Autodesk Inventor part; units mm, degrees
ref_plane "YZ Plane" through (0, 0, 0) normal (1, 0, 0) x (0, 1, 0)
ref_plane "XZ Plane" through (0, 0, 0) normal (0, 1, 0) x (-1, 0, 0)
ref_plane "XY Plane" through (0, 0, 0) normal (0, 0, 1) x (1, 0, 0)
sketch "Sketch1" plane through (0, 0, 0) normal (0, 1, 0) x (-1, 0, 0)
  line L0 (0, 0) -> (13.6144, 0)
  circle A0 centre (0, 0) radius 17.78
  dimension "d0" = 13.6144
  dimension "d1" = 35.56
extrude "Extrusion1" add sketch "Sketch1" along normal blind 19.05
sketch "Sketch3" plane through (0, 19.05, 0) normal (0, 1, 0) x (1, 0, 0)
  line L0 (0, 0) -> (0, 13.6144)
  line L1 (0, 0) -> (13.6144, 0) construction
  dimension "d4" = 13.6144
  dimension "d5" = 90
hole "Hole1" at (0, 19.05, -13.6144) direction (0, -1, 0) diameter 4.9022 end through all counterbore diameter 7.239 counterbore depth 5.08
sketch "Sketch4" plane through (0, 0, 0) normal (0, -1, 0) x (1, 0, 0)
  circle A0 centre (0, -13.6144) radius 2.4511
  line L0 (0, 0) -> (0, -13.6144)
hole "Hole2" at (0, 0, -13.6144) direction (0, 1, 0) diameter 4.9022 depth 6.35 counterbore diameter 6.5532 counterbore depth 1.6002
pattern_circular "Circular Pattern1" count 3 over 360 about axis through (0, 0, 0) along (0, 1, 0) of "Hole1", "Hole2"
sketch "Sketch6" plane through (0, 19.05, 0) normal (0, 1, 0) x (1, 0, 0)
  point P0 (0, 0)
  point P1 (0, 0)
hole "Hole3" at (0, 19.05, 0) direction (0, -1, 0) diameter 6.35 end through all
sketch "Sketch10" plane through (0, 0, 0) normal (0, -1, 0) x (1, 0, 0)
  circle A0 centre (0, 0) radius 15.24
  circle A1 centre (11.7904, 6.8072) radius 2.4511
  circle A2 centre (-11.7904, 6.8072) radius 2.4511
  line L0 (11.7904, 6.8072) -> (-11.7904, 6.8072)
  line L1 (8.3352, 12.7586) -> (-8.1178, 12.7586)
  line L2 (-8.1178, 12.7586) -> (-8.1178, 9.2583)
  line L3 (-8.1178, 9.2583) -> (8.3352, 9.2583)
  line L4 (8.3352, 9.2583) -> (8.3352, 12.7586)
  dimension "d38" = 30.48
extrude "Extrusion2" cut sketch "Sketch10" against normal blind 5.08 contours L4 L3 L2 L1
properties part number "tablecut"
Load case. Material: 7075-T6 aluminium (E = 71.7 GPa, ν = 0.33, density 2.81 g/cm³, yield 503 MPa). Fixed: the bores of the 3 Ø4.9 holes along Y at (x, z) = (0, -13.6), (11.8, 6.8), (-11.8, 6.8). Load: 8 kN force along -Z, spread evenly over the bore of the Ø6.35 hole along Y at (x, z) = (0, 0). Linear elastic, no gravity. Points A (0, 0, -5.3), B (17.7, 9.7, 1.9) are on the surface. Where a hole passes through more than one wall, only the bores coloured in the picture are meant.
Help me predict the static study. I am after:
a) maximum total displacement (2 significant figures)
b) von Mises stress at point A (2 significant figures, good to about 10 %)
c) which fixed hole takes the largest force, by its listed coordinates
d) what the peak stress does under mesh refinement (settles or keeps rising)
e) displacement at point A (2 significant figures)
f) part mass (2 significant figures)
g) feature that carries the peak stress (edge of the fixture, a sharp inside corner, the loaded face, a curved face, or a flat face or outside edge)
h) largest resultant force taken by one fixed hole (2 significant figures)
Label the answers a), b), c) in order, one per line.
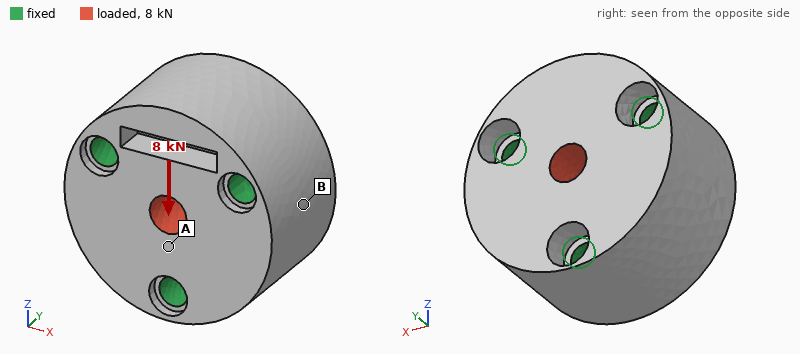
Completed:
a) 5.1 µm
b) 22 MPa
c) (0, -13.6)
d) keeps rising
e) 2.2 µm
f) 46 g
g) edge of the fixture
h) 3.0 kN
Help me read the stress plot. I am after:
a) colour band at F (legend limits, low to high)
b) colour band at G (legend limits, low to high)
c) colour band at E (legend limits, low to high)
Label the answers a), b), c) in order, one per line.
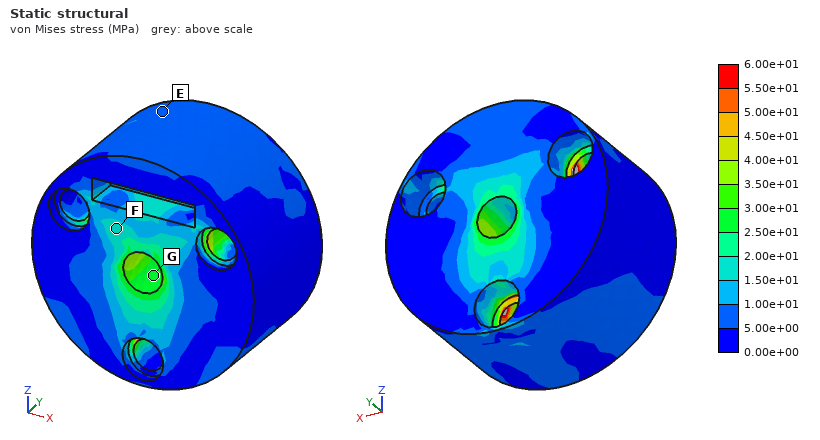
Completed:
a) 1.50e+01 to 2.00e+01 MPa
b) 2.50e+01 to 3.00e+01 MPa
c) 5.00e+00 to 1.00e+01 MPa
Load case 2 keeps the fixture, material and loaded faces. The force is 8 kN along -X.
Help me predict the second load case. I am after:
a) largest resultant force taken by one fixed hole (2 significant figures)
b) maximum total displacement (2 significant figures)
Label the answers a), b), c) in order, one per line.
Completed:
a) 2.8 kN
b) 4.7 µm
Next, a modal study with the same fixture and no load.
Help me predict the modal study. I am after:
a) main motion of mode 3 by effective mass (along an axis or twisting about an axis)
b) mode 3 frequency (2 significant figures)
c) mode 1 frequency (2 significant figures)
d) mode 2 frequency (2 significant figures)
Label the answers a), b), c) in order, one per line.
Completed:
a) along Y
b) 45 kHz
c) 38 kHz
d) 39 kHz
